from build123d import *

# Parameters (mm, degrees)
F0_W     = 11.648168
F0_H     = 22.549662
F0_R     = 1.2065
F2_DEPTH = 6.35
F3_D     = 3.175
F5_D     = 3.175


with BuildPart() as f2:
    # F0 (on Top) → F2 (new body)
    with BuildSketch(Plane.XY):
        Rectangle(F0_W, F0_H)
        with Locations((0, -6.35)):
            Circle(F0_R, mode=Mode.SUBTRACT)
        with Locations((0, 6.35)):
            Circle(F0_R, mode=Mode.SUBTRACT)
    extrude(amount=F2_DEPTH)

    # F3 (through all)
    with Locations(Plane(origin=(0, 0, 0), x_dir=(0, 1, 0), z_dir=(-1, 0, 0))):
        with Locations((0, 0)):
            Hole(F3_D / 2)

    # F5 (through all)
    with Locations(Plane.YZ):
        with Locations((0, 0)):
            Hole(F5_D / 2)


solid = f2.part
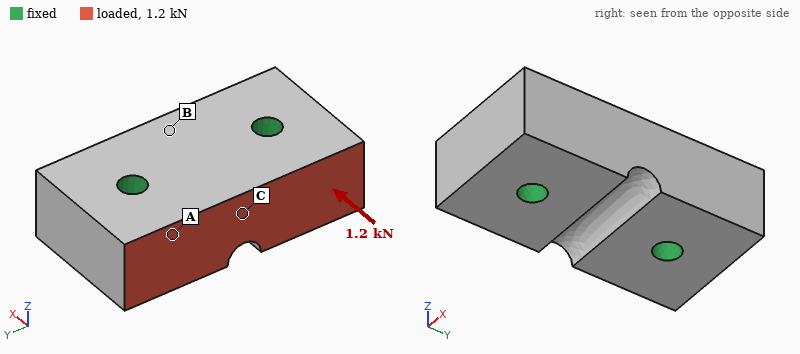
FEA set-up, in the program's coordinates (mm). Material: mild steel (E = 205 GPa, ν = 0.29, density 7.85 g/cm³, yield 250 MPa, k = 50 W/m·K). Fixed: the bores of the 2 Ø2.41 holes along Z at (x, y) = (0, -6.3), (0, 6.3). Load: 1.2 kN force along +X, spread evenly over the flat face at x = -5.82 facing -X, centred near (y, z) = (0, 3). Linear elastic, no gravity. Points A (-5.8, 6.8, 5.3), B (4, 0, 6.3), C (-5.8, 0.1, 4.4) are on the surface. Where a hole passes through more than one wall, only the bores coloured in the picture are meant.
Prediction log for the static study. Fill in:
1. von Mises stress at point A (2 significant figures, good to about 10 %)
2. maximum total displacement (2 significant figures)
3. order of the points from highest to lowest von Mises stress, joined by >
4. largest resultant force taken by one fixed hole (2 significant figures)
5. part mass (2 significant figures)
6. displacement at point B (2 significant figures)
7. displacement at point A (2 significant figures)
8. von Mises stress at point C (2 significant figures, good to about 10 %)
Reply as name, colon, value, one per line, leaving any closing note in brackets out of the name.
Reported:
von Mises stress at point A: 12 MPa
maximum total displacement: 0.43 µm
order of the points from highest to lowest von Mises stress, joined by >: A > C > B
largest resultant force taken by one fixed hole: 600 N
part mass: 12 g
displacement at point B: 0.18 µm
displacement at point A: 0.29 µm
von Mises stress at point C: 7.0 MPa
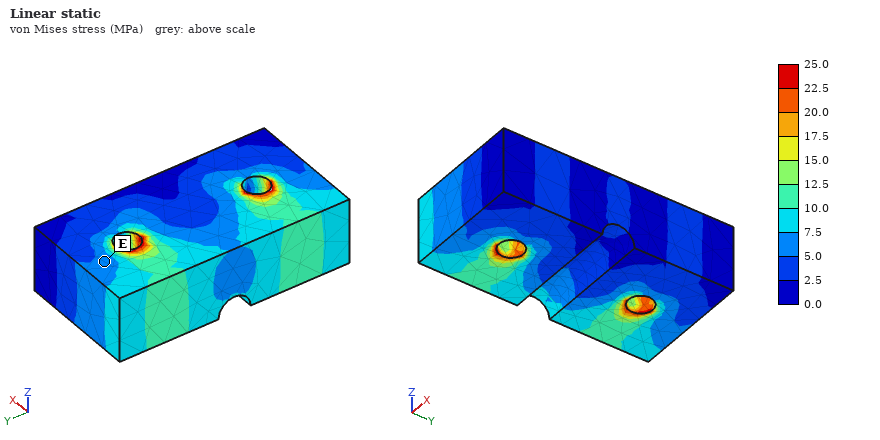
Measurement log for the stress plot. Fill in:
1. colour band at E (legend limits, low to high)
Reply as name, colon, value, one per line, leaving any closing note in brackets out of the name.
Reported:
colour band at E: 5.0 to 7.5 MPa
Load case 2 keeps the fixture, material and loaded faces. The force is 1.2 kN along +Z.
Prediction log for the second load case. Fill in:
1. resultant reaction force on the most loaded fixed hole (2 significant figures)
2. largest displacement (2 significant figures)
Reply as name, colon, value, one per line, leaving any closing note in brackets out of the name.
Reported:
resultant reaction force on the most loaded fixed hole: 600 N
largest displacement: 2.5 µm
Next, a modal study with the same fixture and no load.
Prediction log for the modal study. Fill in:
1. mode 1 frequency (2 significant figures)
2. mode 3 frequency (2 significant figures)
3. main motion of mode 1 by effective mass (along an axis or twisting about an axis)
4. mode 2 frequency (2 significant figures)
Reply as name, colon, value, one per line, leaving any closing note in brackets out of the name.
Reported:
mode 1 frequency: 75 kHz
mode 3 frequency: 86 kHz
main motion of mode 1 by effective mass: twisting about Y
mode 2 frequency: 84 kHz
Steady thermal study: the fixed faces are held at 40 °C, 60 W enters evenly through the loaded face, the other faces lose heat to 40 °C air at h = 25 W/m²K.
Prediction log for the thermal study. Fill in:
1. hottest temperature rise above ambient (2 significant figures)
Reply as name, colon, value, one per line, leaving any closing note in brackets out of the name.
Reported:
hottest temperature rise above ambient: 58 K
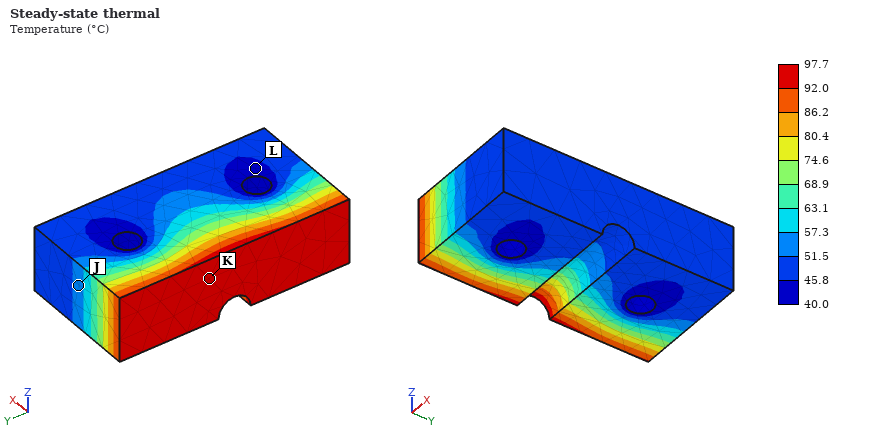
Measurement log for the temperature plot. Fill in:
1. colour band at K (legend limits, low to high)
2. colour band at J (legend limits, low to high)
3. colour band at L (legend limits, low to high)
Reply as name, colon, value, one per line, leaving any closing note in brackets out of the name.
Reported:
colour band at K: 92.0 to 97.7 °C
colour band at J: 51.5 to 57.3 °C
colour band at L: 40.0 to 45.8 °C
